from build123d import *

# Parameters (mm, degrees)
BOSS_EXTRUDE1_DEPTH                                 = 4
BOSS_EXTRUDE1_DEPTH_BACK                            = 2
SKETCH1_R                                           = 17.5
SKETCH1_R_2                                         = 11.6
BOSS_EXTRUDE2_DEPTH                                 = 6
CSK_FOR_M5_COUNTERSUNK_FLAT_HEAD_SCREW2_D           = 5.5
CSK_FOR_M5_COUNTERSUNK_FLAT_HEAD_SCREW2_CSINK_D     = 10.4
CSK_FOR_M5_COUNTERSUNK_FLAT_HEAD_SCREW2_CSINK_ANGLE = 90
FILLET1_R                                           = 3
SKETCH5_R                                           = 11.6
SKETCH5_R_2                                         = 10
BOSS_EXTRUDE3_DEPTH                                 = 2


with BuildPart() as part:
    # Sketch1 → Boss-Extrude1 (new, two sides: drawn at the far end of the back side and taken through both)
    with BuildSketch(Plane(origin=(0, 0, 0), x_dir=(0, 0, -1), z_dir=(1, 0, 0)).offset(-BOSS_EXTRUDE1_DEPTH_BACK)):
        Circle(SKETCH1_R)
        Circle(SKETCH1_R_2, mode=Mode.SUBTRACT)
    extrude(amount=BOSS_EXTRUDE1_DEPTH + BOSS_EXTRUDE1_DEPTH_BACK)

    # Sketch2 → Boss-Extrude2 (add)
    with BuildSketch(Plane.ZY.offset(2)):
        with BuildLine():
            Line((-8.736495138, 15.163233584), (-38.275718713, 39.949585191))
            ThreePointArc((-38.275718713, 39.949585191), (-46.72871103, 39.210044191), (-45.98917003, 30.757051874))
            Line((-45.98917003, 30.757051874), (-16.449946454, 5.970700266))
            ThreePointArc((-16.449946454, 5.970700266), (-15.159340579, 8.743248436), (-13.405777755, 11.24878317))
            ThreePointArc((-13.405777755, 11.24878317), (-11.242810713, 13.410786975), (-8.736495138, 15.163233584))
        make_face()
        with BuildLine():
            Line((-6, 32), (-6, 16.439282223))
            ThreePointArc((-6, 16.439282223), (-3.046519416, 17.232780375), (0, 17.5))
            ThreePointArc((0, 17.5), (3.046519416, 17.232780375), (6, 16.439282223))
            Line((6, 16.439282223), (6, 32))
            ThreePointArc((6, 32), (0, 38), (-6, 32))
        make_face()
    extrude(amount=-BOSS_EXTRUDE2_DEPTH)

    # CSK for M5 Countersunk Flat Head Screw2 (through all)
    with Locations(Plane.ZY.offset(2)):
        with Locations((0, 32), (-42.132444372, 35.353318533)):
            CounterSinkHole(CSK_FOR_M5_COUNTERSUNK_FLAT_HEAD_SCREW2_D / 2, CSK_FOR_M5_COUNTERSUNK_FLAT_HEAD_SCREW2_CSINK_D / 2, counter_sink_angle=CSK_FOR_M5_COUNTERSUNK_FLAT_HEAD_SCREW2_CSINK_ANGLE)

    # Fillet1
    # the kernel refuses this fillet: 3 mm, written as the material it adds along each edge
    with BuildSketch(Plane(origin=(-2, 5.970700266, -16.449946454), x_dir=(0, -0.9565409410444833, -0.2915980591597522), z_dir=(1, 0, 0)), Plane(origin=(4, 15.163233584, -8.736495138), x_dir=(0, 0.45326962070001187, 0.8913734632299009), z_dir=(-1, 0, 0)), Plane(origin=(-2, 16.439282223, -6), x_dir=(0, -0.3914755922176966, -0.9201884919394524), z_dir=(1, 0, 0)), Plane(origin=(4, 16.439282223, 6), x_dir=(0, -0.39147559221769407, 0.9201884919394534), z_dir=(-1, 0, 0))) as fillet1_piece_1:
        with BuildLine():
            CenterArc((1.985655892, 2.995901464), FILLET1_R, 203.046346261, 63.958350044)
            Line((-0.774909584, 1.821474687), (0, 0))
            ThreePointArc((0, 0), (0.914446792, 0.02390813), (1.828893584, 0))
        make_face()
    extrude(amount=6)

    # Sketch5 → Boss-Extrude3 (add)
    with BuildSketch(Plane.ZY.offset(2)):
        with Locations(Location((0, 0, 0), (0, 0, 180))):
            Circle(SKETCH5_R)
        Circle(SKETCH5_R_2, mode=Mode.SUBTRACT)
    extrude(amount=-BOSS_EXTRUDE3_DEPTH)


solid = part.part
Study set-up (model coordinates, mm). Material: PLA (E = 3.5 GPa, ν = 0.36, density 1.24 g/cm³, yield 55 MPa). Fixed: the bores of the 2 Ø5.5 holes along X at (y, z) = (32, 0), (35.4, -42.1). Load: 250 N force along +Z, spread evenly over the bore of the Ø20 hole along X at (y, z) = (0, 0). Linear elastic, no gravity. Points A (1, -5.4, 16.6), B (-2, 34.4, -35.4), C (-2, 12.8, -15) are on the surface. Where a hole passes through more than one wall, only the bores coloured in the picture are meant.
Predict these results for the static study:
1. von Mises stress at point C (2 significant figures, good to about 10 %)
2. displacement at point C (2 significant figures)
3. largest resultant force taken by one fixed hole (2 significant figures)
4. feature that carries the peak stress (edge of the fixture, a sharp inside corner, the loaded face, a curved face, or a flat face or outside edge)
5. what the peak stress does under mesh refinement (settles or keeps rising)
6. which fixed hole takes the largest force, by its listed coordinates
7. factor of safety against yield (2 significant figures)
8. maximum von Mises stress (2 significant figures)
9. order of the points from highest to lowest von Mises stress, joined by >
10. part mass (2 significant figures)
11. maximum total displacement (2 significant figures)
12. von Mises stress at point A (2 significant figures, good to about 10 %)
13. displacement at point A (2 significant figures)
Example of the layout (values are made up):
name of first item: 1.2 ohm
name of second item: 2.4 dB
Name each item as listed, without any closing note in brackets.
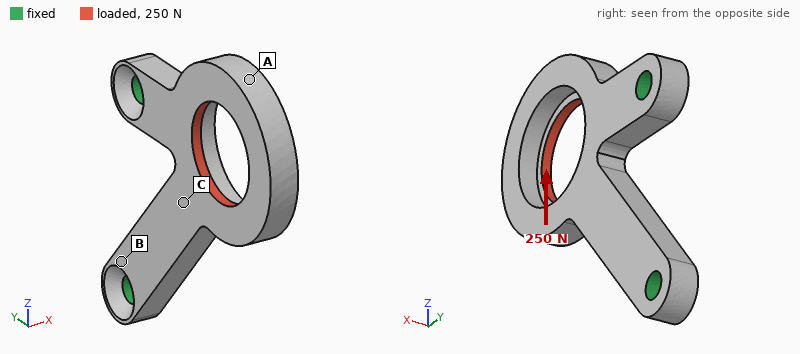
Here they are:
von Mises stress at point C: 3.6 MPa
displacement at point C: 0.061 mm
largest resultant force taken by one fixed hole: 280 N
feature that carries the peak stress: a curved face
what the peak stress does under mesh refinement: settles
which fixed hole takes the largest force, by its listed coordinates: (35.4, -42.1)
factor of safety against yield: 1.9
maximum von Mises stress: 29 MPa
order of the points from highest to lowest von Mises stress, joined by >: A > C > B
part mass: 9.3 g
maximum total displacement: 0.38 mm
von Mises stress at point A: 6.4 MPa
displacement at point A: 0.36 mm
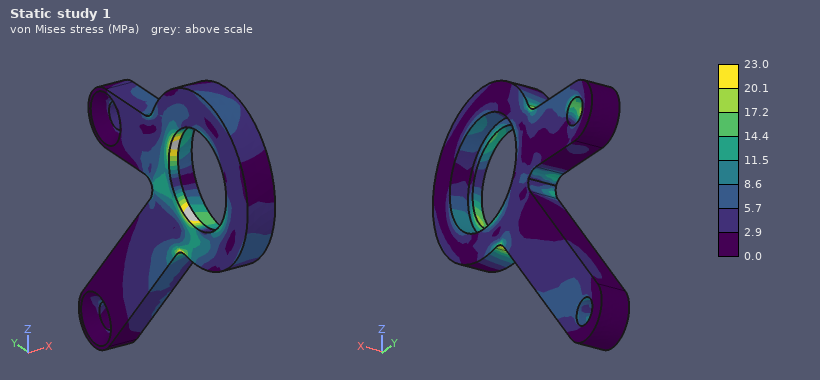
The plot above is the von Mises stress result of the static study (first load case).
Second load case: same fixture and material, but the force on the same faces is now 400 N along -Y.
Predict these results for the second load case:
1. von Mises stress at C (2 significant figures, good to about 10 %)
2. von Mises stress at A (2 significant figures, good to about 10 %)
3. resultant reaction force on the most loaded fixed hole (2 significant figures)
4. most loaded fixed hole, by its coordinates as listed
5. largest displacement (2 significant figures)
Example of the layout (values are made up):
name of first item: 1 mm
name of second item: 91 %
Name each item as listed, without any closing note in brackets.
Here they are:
von Mises stress at C: 6.0 MPa
von Mises stress at A: 4.6 MPa
resultant reaction force on the most loaded fixed hole: 380 N
most loaded fixed hole, by its coordinates as listed: (32, 0)
largest displacement: 0.96 mm
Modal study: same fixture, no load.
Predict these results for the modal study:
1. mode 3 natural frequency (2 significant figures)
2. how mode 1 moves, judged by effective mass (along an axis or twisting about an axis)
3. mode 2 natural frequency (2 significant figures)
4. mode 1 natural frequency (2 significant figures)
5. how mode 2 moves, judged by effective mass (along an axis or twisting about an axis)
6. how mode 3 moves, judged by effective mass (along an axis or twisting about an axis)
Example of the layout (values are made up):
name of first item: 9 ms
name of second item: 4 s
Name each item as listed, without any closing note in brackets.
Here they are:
mode 3 natural frequency: 2100 Hz
how mode 1 moves, judged by effective mass: along X
mode 2 natural frequency: 1600 Hz
mode 1 natural frequency: 610 Hz
how mode 2 moves, judged by effective mass: twisting about Y
how mode 3 moves, judged by effective mass: along Z
